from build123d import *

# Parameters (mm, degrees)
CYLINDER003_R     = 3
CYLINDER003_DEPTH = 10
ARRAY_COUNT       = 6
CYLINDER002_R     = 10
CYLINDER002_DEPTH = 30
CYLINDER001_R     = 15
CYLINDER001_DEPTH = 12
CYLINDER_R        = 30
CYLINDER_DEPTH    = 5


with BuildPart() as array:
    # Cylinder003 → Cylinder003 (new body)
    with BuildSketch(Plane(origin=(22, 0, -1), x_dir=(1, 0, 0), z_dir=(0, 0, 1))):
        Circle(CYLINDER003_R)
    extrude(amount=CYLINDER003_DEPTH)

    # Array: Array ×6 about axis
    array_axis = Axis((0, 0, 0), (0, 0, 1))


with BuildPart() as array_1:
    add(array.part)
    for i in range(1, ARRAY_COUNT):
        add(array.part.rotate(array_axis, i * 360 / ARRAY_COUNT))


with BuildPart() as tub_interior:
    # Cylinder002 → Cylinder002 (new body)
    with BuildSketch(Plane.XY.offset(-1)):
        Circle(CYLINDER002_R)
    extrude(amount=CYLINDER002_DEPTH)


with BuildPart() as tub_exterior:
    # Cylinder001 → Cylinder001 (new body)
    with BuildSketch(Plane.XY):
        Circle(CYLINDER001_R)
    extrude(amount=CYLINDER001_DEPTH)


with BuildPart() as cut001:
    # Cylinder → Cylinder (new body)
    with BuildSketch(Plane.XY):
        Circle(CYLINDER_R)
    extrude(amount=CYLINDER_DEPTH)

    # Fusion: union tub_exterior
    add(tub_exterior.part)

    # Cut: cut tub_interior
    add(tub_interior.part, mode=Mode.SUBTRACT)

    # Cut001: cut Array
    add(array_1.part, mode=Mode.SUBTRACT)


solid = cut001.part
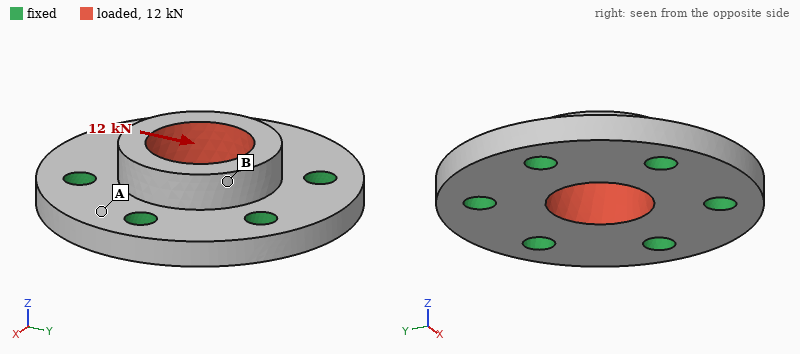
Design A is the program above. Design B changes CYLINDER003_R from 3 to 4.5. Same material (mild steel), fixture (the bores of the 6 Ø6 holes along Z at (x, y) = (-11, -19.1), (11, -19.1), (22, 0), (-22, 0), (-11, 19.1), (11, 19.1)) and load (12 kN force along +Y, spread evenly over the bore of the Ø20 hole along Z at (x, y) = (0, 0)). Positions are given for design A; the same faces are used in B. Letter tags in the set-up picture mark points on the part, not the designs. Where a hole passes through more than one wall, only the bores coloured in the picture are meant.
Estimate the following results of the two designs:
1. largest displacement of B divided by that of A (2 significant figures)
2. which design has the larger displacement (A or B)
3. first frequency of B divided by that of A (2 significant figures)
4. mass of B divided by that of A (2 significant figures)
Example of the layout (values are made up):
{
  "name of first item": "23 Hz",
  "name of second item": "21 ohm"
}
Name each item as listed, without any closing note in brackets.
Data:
{
  "largest displacement of B divided by that of A": "0.92",
  "which design has the larger displacement": "A",
  "first frequency of B divided by that of A": "1.3",
  "mass of B divided by that of A": "0.93"
}
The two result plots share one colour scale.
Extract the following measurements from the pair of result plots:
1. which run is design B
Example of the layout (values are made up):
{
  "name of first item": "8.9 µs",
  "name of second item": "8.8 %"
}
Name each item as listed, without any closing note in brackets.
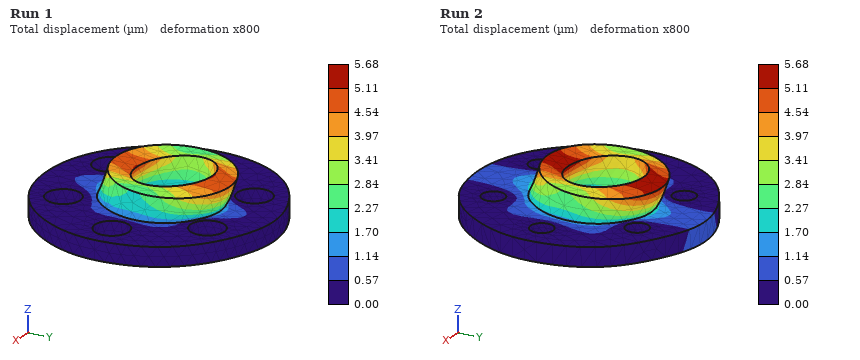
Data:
{
  "which run is design B": "Run 1"
}
